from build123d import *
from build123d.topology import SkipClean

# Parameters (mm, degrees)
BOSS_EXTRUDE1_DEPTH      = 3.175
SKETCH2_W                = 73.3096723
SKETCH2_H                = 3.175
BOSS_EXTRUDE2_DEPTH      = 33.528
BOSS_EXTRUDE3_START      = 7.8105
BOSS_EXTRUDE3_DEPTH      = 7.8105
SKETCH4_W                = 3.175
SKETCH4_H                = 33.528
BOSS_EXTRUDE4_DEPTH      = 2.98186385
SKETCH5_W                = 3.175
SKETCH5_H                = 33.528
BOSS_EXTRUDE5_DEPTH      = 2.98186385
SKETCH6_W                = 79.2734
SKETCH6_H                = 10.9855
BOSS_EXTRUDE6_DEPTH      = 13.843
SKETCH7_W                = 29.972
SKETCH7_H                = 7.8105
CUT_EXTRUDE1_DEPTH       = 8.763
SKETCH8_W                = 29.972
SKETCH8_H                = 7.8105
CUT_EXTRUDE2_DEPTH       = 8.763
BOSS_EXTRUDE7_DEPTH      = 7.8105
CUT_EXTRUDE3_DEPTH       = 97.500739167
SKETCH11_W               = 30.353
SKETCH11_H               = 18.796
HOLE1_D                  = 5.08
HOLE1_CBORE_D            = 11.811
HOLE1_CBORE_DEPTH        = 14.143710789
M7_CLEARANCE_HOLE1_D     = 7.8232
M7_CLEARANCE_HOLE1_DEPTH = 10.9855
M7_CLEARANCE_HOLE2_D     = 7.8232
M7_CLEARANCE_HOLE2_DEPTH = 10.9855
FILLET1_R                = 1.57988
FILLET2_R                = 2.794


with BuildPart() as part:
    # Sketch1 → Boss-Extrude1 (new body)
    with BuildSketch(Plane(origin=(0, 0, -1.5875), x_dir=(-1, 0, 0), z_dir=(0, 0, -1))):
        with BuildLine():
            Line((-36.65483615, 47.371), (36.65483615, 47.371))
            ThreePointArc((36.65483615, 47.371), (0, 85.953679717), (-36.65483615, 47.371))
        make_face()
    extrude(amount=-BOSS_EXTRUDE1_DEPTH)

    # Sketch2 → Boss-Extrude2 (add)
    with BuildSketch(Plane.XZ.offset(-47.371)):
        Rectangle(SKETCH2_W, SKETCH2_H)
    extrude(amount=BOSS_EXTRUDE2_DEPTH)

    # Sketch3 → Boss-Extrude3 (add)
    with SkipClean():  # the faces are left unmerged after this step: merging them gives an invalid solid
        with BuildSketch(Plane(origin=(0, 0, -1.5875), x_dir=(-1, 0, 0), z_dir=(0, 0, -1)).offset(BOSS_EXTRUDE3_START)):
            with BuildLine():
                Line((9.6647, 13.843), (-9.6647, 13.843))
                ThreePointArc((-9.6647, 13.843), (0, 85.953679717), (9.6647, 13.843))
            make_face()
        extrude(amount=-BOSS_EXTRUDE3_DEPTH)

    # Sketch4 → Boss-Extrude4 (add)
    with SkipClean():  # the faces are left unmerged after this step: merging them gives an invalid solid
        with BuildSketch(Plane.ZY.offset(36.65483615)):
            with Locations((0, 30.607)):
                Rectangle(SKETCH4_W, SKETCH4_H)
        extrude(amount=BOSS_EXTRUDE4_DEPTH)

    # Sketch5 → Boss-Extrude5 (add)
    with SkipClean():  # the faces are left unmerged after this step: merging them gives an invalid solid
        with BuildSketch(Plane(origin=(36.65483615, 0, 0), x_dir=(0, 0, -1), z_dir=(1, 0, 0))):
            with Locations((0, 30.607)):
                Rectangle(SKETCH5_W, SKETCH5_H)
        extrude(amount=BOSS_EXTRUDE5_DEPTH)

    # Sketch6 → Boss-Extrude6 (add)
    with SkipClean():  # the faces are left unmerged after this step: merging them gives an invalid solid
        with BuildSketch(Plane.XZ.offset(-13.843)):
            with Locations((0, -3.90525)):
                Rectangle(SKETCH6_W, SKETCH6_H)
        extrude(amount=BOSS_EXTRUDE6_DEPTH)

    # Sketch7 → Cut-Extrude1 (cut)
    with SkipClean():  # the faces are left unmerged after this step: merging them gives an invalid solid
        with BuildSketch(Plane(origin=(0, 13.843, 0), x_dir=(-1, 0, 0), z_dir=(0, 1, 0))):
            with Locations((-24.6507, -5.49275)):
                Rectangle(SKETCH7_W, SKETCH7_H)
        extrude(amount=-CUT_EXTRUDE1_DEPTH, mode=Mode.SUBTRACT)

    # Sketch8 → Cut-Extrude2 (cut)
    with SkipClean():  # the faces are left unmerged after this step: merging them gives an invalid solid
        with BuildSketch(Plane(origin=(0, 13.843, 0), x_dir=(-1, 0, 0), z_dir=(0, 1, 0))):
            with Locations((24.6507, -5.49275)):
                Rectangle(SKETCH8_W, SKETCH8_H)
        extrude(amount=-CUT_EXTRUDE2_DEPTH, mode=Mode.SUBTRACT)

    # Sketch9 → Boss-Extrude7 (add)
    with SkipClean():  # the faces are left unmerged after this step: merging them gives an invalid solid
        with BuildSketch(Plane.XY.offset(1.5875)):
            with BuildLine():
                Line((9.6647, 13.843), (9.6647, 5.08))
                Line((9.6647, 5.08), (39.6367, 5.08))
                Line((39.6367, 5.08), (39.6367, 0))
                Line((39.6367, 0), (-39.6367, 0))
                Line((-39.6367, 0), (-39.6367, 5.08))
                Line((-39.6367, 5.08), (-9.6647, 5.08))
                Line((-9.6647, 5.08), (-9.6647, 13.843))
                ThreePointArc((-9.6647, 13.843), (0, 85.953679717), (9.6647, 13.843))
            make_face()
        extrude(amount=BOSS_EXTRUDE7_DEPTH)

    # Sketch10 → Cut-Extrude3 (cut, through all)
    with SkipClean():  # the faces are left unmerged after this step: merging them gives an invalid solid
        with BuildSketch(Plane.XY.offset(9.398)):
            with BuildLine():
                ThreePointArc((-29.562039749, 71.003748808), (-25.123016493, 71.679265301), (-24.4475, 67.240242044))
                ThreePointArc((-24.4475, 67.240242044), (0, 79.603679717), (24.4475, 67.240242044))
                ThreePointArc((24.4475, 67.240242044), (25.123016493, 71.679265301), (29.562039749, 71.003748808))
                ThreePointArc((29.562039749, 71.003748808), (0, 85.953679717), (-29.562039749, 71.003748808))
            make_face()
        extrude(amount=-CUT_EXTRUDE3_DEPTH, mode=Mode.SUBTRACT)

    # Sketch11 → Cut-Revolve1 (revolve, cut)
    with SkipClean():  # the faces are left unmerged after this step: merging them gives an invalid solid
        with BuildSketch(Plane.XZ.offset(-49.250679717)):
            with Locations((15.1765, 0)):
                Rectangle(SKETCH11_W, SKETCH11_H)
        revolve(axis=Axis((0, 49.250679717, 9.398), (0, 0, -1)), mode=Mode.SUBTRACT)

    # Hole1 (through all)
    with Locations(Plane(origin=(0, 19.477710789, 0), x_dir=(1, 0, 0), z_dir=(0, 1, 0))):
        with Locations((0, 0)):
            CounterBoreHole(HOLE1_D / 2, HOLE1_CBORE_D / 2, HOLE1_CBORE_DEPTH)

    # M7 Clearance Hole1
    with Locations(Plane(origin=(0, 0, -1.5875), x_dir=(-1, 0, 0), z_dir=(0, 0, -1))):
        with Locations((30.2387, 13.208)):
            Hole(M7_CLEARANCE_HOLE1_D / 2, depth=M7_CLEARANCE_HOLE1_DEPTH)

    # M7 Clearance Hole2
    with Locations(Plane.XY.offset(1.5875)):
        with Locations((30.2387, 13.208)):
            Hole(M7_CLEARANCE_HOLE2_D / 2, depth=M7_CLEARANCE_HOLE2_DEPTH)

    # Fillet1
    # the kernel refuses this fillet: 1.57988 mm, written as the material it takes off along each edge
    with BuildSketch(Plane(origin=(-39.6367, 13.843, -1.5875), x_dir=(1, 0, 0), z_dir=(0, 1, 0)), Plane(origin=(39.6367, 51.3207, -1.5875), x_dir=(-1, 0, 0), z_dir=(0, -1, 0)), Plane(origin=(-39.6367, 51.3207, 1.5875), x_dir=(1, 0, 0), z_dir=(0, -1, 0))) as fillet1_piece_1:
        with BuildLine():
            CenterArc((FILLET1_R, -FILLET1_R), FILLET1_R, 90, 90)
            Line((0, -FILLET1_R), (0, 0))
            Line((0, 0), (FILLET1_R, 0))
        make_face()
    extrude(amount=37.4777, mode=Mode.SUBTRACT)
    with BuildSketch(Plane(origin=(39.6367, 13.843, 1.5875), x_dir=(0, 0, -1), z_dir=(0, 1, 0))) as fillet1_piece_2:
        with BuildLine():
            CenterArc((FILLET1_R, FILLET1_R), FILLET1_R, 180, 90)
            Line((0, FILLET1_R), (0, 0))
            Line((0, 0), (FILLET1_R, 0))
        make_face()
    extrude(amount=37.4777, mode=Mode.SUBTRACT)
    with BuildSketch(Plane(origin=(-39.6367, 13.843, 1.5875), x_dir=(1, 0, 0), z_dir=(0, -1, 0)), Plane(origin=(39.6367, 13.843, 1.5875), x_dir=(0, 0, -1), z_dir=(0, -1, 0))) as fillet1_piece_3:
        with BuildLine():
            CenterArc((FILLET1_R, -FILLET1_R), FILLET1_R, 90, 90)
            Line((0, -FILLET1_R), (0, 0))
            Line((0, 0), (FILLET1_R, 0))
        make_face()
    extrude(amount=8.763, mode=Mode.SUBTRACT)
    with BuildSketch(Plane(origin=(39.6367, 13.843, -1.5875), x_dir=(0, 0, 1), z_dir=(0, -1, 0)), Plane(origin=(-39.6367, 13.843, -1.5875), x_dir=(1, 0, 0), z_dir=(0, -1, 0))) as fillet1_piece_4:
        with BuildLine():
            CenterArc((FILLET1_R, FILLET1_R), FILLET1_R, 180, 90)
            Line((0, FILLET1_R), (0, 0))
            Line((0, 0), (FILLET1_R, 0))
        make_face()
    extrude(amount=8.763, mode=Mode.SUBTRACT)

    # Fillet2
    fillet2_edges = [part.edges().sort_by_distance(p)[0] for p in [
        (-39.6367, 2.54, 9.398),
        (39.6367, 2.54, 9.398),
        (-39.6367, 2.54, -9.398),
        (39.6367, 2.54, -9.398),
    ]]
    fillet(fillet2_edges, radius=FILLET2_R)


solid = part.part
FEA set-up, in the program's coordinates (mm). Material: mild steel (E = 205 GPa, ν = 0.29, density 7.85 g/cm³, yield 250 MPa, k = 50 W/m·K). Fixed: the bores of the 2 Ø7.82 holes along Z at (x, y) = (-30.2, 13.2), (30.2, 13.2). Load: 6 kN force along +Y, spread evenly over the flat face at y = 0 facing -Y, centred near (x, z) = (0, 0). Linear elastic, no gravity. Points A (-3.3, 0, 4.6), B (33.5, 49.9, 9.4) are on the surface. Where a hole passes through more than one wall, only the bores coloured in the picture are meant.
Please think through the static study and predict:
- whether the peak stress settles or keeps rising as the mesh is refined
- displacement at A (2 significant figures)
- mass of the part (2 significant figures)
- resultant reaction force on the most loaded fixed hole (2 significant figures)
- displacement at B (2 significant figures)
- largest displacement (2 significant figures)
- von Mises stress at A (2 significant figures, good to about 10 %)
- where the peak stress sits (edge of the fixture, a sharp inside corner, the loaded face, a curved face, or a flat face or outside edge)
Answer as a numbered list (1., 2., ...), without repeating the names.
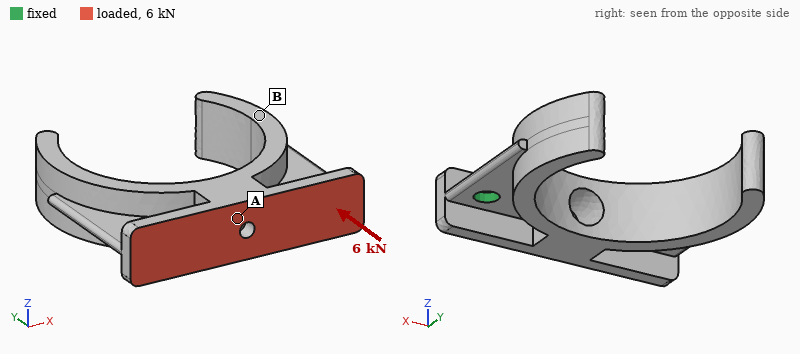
1. keeps rising
2. 8.5 µm
3. 240 g
4. 3.2 kN
5. 11 µm
6. 18 µm
7. 27 MPa
8. edge of the fixture
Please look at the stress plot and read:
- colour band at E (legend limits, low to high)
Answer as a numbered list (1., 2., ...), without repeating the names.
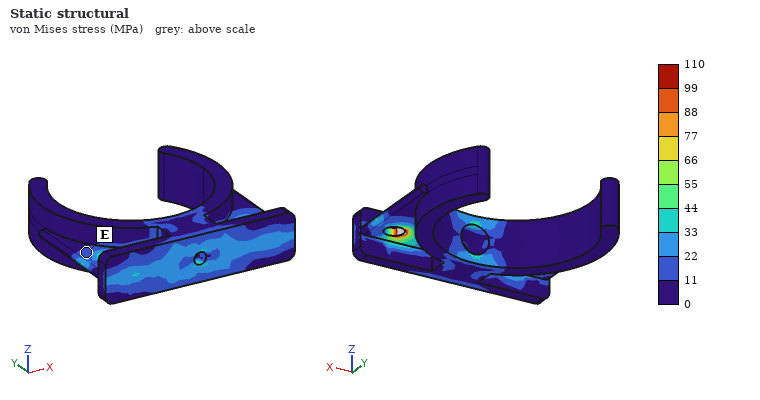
1. 11 to 22 MPa
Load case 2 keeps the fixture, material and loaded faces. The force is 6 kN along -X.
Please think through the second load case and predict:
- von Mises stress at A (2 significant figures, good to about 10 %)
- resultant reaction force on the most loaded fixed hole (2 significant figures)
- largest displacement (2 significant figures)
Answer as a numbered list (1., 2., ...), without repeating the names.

1. 7.6 MPa
2. 3.2 kN
3. 5.7 µm
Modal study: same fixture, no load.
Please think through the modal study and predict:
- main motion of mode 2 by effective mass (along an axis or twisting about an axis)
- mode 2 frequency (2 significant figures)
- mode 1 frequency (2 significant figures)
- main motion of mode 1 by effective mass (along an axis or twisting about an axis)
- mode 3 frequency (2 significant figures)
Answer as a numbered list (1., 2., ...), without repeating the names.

1. twisting about Y
2. 2000 Hz
3. 1300 Hz
4. along Z
5. 2900 Hz
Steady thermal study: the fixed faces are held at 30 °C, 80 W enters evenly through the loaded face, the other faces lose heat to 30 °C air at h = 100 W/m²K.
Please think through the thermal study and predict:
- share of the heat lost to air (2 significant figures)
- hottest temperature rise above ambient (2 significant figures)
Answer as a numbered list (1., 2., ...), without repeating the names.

1. 38 %
2. 60 K
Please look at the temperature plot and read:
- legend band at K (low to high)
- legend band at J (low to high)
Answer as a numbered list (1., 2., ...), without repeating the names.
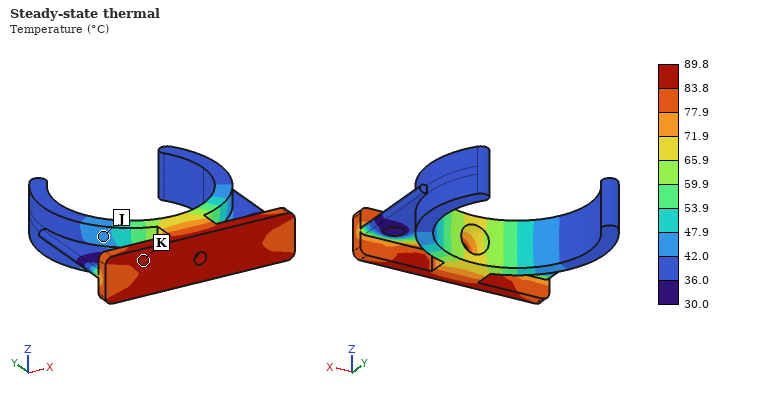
1. 83.8 to 89.8 °C
2. 42.0 to 47.9 °C
